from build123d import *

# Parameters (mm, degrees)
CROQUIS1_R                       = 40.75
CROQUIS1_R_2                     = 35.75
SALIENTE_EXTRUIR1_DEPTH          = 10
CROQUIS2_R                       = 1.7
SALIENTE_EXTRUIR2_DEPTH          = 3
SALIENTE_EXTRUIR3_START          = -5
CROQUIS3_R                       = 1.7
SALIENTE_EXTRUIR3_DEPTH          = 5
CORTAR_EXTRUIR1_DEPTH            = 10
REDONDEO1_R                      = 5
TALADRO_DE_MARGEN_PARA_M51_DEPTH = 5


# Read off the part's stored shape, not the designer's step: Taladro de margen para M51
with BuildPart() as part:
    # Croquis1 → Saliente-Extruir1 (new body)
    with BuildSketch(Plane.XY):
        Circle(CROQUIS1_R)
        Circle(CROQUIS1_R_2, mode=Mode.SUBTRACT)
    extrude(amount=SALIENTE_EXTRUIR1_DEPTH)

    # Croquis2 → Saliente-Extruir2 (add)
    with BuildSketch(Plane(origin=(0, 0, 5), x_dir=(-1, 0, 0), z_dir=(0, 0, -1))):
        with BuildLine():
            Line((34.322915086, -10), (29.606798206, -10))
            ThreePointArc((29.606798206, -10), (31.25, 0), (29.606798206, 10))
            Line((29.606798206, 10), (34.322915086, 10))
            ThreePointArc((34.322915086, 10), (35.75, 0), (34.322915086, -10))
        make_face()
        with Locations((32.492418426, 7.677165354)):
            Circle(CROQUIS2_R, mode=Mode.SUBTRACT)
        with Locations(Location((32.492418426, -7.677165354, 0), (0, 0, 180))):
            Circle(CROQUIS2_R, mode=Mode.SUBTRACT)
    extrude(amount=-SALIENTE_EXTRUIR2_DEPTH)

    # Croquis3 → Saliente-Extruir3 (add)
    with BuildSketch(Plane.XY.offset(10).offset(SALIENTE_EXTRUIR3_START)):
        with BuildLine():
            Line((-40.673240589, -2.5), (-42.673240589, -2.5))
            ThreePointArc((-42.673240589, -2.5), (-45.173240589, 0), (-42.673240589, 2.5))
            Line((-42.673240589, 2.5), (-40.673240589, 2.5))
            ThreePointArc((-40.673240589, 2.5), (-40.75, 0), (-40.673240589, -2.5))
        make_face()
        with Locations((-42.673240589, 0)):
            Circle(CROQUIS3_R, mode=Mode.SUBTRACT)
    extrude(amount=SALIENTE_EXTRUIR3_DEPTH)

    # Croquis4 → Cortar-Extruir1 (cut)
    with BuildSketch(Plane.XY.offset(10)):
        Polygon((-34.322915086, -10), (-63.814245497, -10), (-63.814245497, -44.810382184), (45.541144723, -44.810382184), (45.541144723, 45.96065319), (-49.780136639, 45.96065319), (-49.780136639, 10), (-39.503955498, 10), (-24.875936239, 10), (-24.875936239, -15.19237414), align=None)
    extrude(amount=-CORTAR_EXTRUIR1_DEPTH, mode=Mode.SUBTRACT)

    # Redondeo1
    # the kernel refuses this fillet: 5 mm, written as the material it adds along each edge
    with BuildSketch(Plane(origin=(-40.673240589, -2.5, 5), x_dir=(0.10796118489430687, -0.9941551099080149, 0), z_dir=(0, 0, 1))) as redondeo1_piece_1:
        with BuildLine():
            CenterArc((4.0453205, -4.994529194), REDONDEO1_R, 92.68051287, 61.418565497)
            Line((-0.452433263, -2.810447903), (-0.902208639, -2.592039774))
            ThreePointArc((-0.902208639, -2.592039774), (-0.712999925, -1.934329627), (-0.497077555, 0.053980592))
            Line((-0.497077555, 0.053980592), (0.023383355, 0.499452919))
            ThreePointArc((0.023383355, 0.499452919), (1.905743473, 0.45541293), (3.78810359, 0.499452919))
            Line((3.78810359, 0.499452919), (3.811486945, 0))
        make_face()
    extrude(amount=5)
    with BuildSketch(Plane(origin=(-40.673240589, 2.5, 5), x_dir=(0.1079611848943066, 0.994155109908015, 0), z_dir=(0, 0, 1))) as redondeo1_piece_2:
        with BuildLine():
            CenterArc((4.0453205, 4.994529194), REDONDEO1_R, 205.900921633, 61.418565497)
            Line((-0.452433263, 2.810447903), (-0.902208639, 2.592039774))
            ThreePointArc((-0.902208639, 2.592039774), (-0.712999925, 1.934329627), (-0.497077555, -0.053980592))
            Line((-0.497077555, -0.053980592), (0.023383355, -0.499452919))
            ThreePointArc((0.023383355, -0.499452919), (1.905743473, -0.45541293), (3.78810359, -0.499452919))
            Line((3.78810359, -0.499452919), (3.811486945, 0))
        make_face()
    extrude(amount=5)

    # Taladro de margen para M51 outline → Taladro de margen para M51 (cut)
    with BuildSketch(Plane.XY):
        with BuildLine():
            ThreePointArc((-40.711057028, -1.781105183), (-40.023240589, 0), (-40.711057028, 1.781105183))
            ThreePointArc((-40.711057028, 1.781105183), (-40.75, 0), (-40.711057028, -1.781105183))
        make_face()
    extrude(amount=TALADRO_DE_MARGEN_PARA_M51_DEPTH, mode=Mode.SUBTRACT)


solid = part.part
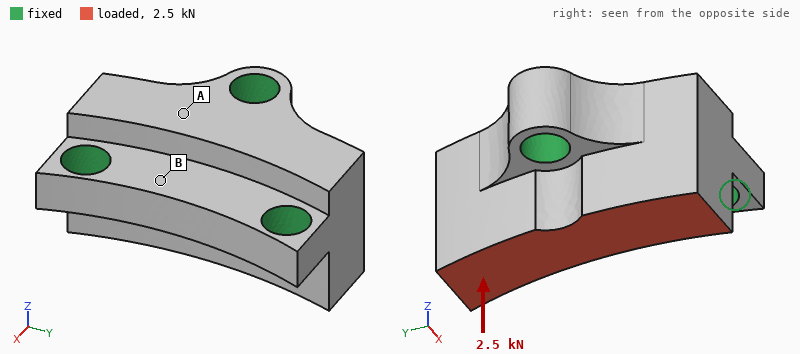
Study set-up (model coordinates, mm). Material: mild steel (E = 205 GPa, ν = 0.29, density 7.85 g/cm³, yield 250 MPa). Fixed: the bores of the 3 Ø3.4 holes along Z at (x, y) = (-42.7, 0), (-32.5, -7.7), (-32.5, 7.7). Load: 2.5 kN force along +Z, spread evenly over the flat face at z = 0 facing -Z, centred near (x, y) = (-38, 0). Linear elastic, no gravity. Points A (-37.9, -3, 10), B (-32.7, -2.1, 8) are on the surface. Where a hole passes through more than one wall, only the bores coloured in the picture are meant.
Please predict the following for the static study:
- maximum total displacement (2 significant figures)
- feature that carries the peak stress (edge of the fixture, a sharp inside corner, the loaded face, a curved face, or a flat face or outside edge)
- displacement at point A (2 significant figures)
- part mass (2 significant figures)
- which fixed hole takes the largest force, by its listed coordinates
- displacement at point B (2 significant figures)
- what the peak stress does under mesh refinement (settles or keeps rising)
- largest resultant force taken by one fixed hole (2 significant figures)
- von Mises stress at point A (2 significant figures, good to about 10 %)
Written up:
3.2 µm
edge of the fixture
1.2 µm
10 g
(-42.7, 0)
0.68 µm
keeps rising
1.3 kN
30 MPa
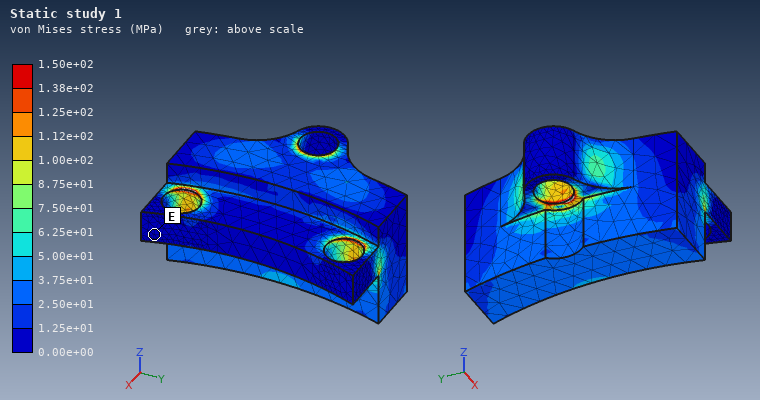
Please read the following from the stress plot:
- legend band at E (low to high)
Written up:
0.00e+00 to 1.25e+01 MPa
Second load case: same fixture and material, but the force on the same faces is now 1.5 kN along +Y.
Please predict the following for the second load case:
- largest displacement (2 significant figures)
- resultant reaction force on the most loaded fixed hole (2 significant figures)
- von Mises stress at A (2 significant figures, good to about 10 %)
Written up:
6.0 µm
700 N
21 MPa
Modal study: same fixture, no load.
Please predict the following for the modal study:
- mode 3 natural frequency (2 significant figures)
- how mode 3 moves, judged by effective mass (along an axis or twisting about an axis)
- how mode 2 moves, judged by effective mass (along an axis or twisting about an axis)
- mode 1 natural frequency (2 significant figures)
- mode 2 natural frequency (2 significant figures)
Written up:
71 kHz
along Z
along X
49 kHz
56 kHz
